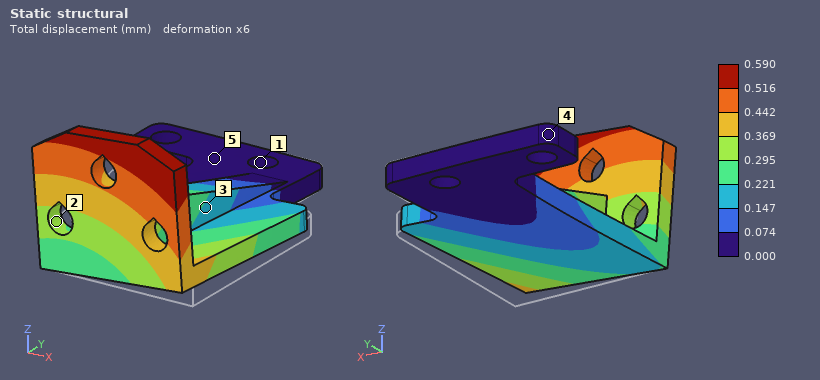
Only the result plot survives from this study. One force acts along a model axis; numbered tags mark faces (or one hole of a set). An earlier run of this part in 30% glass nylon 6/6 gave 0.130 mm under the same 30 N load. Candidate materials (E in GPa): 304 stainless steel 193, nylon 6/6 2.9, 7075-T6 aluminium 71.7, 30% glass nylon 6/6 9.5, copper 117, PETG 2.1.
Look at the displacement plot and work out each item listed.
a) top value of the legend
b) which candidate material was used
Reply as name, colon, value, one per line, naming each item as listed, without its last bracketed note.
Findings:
top value of the legend: 0.590 mm
which candidate material was used: PETG
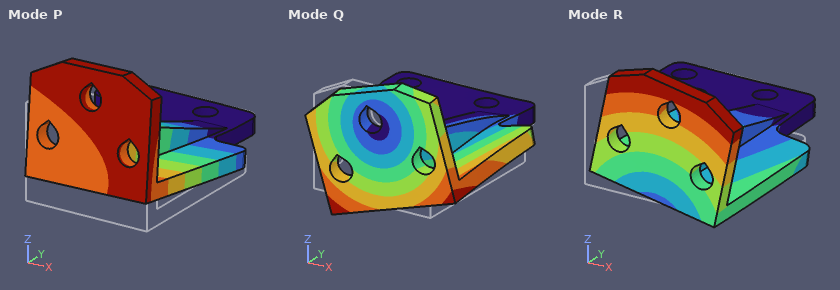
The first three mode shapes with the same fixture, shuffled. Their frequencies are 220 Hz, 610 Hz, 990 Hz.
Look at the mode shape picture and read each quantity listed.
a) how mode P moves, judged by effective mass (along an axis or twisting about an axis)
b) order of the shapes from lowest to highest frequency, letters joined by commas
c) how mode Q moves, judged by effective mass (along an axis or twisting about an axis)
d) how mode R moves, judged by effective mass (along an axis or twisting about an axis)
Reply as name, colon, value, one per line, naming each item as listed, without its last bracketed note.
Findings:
how mode P moves, judged by effective mass: along Z
order of the shapes from lowest to highest frequency, letters joined by commas: P, R, Q
how mode Q moves, judged by effective mass: along X
how mode R moves, judged by effective mass: along X
